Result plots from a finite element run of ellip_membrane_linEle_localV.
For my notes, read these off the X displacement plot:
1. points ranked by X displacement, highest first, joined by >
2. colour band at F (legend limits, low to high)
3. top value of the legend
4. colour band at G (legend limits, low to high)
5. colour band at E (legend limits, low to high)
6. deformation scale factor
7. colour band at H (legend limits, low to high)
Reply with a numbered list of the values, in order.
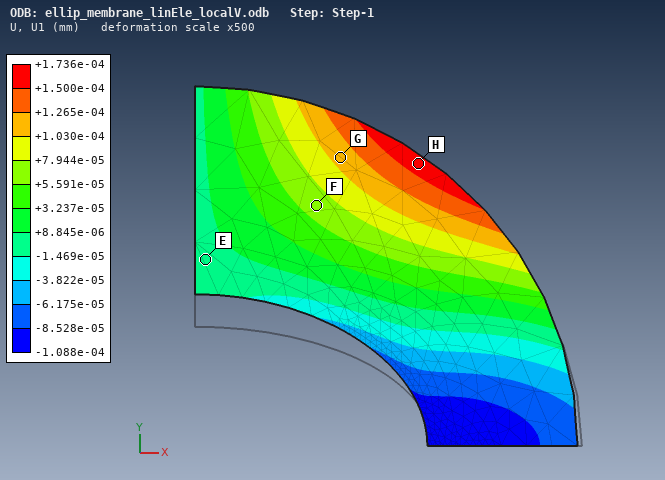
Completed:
1. H > G > F > E
2. +5.591e-05 to +7.944e-05 mm
3. +1.736e-04 mm
4. +1.030e-04 to +1.265e-04 mm
5. -1.469e-05 to +8.845e-06 mm
6. 500
7. +1.500e-04 to +1.736e-04 mm
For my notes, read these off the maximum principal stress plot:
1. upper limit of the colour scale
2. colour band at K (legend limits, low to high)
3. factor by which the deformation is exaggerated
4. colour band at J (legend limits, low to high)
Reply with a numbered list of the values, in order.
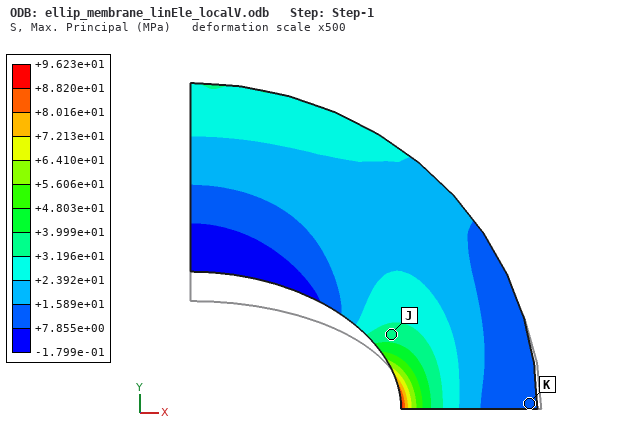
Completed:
1. +9.623e+01 MPa
2. +7.855e+00 to +1.589e+01 MPa
3. 500
4. +3.196e+01 to +3.999e+01 MPa
